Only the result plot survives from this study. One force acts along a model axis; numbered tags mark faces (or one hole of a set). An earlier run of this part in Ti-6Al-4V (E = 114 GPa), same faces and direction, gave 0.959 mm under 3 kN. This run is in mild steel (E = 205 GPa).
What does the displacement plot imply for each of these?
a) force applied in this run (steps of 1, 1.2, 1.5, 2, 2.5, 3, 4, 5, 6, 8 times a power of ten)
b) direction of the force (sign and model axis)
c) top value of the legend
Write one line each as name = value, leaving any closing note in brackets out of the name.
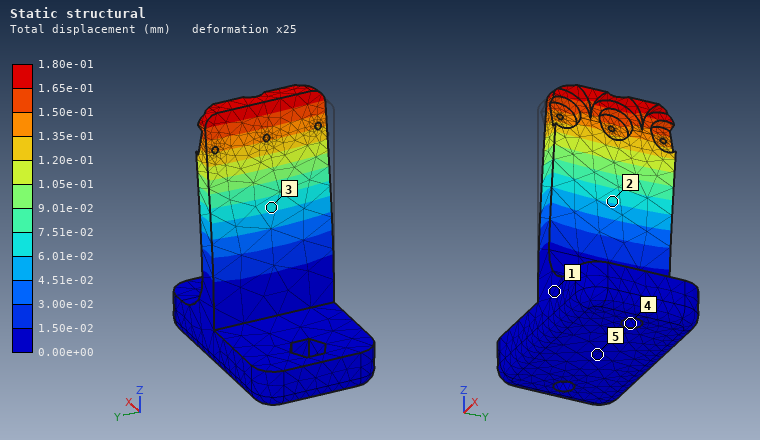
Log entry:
force applied in this run = 1 kN
direction of the force = +X
top value of the legend = 1.80e-01 mm
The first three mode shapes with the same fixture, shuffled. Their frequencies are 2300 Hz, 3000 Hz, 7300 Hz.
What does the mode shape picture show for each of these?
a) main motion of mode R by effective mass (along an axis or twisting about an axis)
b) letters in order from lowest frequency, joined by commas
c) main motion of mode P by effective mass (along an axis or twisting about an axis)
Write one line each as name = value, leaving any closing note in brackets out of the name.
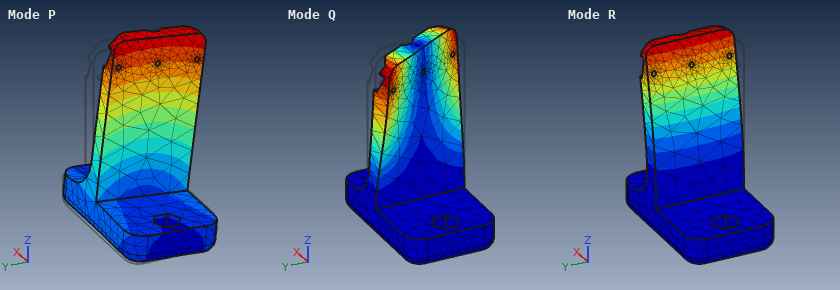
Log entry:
main motion of mode R by effective mass = along X
letters in order from lowest frequency, joined by commas = R, P, Q
main motion of mode P by effective mass = along Y
